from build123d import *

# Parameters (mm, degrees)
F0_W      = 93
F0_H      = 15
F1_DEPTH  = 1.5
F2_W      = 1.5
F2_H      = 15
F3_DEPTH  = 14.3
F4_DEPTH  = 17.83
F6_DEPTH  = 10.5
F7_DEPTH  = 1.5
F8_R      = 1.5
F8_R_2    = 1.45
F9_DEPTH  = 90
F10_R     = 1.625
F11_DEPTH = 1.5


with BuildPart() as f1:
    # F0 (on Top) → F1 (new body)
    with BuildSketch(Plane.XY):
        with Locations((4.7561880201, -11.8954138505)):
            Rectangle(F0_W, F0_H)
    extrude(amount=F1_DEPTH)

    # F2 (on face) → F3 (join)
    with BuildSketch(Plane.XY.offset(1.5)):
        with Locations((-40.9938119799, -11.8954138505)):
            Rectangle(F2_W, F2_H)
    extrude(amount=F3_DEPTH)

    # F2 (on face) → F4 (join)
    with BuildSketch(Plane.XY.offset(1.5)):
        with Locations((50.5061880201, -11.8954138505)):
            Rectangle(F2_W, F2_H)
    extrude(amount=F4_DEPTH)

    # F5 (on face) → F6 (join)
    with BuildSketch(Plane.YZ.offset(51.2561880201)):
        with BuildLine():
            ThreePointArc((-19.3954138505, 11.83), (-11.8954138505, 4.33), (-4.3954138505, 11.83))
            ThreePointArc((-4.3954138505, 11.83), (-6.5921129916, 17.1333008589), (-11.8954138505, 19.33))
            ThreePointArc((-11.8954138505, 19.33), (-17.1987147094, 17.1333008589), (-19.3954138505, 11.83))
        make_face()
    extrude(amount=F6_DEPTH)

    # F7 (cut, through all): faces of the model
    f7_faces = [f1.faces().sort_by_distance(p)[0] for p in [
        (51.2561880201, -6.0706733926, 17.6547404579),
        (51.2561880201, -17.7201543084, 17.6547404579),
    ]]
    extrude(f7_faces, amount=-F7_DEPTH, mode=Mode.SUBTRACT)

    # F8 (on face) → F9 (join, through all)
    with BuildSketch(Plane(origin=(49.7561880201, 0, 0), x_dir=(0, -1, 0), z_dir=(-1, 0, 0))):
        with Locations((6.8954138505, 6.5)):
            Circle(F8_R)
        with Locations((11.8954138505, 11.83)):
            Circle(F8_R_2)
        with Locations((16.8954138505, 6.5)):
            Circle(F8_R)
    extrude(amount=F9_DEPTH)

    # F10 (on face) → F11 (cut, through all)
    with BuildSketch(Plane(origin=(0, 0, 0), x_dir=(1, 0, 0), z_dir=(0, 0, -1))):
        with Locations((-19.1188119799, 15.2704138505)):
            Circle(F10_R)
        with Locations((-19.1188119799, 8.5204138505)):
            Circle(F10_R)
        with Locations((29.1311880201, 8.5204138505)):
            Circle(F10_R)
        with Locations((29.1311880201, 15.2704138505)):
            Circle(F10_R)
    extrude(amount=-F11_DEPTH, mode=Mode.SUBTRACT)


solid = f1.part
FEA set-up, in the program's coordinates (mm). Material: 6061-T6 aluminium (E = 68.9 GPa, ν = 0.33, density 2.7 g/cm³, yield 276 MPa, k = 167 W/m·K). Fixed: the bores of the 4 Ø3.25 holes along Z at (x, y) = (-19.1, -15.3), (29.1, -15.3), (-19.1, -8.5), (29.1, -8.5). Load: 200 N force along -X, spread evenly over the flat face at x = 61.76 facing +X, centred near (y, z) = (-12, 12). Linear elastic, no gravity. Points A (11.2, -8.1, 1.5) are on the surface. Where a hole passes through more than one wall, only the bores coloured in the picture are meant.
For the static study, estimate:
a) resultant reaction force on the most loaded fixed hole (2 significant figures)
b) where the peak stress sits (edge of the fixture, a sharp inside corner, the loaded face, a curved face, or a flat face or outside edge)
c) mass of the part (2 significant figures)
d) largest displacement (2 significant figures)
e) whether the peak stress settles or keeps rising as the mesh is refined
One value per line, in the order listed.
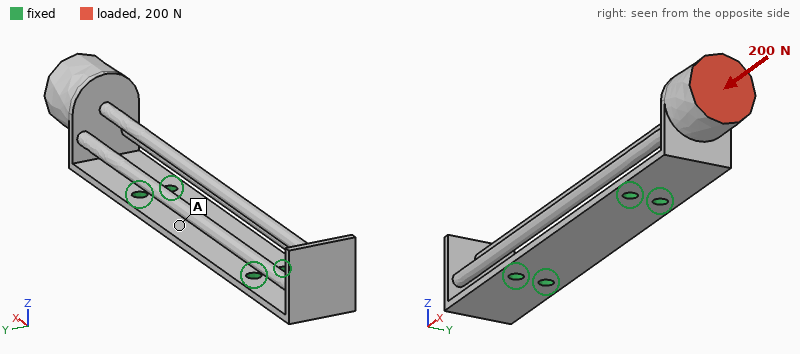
60 N
edge of the fixture
17 g
0.78 mm
keeps rising
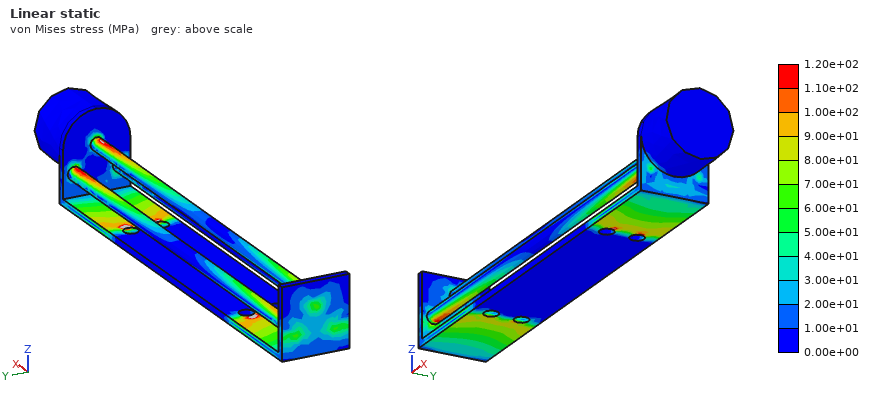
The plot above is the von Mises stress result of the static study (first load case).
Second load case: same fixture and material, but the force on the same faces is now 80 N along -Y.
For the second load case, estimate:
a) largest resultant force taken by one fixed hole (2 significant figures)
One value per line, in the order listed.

260 N
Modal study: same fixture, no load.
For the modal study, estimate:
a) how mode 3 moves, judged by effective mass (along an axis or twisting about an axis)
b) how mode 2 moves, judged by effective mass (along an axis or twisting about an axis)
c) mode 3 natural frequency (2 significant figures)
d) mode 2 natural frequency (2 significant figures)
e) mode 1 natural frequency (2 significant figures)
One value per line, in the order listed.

along Z
along Y
1100 Hz
860 Hz
700 Hz
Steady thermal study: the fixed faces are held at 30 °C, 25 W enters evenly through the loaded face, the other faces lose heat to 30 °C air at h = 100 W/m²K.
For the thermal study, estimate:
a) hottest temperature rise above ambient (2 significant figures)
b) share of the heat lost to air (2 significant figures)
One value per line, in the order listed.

84 K
60 %
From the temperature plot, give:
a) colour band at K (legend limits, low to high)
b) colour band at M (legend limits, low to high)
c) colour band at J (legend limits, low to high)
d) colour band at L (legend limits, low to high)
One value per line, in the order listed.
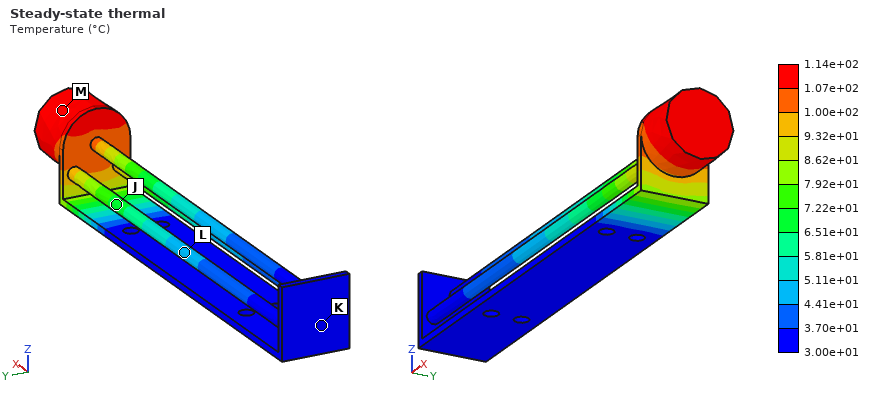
3.00e+01 to 3.70e+01 °C
1.07e+02 to 1.14e+02 °C
6.51e+01 to 7.22e+01 °C
4.41e+01 to 5.11e+01 °C
